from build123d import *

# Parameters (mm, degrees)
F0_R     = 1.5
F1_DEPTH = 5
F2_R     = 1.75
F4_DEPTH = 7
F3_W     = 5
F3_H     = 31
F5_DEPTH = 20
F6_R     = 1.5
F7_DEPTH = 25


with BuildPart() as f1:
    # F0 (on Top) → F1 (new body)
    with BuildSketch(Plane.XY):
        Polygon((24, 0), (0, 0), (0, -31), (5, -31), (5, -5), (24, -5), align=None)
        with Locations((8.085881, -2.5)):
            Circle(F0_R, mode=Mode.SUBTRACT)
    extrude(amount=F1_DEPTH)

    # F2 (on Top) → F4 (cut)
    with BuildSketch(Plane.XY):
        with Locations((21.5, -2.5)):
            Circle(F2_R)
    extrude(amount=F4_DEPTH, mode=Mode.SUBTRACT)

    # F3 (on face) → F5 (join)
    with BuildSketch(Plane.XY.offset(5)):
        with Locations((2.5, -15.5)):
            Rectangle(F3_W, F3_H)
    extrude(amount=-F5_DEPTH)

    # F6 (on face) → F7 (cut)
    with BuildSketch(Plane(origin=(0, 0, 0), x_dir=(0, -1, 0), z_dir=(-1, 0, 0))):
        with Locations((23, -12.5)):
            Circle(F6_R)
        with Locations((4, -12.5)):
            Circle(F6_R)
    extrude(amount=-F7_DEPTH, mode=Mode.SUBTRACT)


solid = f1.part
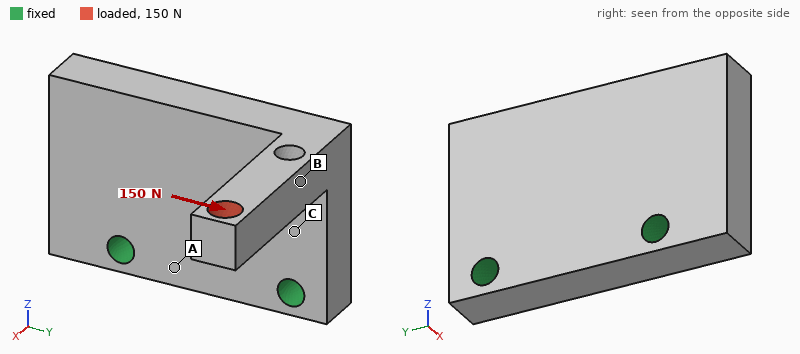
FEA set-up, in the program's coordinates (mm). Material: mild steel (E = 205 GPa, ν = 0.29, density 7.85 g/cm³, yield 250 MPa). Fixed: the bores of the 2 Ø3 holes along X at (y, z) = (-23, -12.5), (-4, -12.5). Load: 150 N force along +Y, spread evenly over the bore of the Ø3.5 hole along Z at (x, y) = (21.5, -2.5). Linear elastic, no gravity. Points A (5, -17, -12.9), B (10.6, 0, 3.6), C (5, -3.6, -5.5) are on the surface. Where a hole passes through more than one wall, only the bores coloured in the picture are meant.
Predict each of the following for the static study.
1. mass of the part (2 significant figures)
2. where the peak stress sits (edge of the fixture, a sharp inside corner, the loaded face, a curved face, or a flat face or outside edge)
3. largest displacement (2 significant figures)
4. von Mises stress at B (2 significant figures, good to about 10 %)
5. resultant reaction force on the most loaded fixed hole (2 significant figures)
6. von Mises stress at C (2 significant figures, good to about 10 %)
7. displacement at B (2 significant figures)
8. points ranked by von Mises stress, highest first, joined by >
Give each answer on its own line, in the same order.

27 g
a flat face or outside edge
64 µm
75 MPa
180 N
39 MPa
19 µm
B > C > A
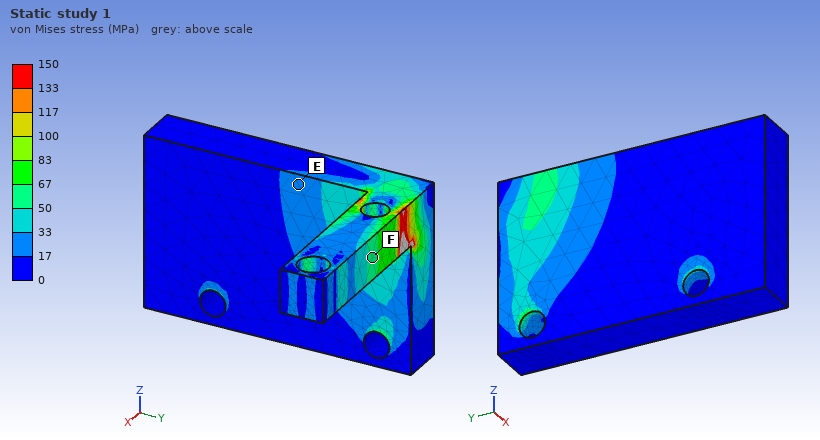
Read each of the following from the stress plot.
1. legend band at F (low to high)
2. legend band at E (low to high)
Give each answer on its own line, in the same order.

50 to 67 MPa
17 to 33 MPa
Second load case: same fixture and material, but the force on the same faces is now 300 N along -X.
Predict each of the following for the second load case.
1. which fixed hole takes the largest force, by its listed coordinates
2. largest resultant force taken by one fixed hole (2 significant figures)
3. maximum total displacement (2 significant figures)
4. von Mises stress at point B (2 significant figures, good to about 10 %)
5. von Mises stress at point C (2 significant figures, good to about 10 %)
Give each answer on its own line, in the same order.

(-4, -12.5)
300 N
28 µm
23 MPa
38 MPa
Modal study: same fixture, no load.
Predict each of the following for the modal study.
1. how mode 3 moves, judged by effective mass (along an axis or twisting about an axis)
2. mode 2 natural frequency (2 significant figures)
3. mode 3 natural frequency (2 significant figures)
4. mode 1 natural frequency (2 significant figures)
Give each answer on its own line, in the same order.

along X
7600 Hz
11 kHz
6200 Hz
